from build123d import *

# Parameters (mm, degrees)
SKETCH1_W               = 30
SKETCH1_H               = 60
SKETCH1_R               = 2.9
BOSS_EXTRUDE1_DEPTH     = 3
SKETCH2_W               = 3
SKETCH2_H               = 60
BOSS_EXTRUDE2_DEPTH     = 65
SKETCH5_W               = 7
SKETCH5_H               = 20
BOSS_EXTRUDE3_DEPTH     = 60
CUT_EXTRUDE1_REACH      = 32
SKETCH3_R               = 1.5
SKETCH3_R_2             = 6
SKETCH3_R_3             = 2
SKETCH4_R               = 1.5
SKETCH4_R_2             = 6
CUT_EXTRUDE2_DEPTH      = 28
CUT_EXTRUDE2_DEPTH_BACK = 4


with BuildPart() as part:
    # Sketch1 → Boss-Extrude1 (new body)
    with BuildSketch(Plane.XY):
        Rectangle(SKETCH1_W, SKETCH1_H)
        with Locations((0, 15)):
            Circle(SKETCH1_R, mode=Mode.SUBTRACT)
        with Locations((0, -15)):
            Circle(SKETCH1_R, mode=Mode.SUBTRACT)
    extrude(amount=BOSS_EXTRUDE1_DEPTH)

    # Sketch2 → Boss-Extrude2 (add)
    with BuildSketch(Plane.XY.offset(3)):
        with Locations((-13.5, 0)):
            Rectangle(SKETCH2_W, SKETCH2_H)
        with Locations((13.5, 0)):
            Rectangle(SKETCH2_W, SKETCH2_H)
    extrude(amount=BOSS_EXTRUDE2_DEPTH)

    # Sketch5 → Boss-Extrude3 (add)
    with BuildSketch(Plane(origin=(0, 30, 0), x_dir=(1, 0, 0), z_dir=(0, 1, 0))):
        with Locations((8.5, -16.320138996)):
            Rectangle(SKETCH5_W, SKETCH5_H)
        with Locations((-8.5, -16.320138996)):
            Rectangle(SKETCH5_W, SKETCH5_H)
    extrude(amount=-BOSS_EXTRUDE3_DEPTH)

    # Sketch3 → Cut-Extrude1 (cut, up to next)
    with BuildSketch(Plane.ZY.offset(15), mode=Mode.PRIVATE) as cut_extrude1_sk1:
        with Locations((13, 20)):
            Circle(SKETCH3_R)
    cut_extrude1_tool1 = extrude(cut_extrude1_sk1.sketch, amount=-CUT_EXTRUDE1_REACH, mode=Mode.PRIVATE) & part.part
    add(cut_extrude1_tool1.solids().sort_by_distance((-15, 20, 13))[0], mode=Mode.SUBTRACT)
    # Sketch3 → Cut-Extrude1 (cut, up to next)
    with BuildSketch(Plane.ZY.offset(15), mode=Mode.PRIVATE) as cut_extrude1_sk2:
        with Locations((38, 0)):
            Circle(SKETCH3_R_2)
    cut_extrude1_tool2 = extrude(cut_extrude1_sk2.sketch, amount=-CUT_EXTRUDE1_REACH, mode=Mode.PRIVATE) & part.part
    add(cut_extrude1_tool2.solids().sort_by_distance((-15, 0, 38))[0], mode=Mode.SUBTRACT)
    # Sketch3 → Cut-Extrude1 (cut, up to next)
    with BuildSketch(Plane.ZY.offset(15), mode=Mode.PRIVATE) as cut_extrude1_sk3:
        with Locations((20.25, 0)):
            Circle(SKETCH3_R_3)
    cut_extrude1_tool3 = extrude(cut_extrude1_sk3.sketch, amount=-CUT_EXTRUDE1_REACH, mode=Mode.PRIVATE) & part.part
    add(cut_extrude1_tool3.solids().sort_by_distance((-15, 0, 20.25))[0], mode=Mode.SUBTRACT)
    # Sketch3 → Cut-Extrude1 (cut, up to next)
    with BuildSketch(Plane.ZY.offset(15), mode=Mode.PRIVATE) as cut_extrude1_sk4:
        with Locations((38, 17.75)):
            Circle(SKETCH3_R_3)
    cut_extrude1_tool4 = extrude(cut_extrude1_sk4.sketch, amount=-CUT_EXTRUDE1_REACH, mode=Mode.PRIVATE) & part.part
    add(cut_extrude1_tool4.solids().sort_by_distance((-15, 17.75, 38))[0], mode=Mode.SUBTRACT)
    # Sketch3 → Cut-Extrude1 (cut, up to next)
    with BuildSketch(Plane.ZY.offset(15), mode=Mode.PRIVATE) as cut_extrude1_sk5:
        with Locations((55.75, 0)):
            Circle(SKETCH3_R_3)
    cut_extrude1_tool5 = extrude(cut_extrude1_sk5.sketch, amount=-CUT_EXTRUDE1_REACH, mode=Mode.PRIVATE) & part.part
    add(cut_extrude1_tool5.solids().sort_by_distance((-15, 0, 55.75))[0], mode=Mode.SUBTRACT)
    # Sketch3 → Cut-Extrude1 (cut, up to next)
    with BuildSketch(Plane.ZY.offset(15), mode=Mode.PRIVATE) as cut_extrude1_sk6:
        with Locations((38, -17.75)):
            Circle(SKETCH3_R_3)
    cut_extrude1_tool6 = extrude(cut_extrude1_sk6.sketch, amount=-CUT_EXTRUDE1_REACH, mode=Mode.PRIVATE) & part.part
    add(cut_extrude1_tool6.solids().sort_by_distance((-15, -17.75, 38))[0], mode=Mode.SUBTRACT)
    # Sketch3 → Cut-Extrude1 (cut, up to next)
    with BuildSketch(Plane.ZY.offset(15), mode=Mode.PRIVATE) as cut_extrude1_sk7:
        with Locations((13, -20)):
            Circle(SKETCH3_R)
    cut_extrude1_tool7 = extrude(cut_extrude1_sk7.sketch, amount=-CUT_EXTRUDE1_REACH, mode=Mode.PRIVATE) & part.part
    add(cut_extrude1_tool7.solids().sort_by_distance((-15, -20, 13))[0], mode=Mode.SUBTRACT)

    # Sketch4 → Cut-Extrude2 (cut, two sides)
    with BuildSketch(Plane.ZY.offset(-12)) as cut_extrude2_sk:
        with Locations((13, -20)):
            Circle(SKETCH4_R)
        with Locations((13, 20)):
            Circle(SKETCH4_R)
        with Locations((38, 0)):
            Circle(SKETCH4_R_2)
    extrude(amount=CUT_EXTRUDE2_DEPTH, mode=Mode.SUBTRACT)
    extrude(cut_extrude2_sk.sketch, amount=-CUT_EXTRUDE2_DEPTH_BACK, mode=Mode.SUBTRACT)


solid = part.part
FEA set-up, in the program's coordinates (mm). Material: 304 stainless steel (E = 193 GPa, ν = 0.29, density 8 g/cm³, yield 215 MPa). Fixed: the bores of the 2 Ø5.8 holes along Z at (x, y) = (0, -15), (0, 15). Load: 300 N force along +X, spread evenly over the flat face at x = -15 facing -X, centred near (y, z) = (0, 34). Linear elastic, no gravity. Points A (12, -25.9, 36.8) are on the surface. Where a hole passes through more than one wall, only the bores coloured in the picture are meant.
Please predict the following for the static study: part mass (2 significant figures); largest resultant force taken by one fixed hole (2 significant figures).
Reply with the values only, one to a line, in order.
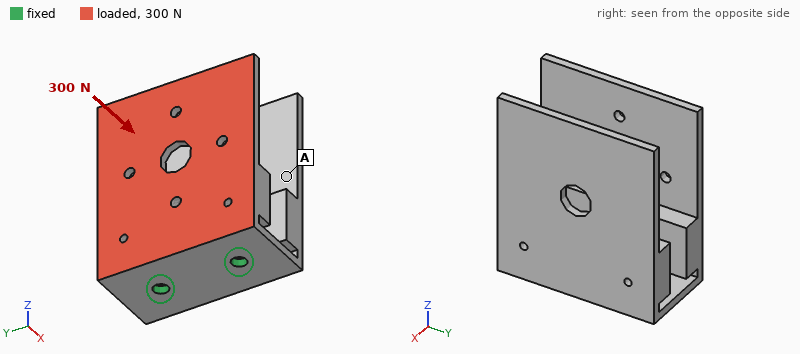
350 g
150 N
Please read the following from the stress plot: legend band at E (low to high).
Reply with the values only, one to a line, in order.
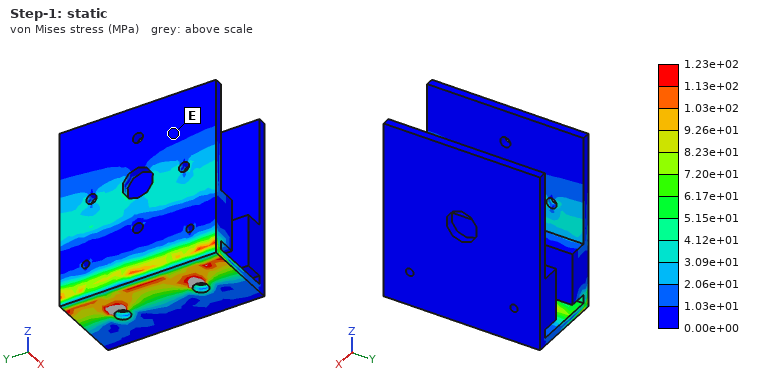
0.00e+00 to 1.03e+01 MPa
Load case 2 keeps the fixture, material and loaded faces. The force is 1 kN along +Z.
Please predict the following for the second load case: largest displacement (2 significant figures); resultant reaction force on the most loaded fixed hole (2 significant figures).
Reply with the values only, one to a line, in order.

0.30 mm
500 N
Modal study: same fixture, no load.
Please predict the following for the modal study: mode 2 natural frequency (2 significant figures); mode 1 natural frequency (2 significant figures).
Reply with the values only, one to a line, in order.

490 Hz
470 Hz
